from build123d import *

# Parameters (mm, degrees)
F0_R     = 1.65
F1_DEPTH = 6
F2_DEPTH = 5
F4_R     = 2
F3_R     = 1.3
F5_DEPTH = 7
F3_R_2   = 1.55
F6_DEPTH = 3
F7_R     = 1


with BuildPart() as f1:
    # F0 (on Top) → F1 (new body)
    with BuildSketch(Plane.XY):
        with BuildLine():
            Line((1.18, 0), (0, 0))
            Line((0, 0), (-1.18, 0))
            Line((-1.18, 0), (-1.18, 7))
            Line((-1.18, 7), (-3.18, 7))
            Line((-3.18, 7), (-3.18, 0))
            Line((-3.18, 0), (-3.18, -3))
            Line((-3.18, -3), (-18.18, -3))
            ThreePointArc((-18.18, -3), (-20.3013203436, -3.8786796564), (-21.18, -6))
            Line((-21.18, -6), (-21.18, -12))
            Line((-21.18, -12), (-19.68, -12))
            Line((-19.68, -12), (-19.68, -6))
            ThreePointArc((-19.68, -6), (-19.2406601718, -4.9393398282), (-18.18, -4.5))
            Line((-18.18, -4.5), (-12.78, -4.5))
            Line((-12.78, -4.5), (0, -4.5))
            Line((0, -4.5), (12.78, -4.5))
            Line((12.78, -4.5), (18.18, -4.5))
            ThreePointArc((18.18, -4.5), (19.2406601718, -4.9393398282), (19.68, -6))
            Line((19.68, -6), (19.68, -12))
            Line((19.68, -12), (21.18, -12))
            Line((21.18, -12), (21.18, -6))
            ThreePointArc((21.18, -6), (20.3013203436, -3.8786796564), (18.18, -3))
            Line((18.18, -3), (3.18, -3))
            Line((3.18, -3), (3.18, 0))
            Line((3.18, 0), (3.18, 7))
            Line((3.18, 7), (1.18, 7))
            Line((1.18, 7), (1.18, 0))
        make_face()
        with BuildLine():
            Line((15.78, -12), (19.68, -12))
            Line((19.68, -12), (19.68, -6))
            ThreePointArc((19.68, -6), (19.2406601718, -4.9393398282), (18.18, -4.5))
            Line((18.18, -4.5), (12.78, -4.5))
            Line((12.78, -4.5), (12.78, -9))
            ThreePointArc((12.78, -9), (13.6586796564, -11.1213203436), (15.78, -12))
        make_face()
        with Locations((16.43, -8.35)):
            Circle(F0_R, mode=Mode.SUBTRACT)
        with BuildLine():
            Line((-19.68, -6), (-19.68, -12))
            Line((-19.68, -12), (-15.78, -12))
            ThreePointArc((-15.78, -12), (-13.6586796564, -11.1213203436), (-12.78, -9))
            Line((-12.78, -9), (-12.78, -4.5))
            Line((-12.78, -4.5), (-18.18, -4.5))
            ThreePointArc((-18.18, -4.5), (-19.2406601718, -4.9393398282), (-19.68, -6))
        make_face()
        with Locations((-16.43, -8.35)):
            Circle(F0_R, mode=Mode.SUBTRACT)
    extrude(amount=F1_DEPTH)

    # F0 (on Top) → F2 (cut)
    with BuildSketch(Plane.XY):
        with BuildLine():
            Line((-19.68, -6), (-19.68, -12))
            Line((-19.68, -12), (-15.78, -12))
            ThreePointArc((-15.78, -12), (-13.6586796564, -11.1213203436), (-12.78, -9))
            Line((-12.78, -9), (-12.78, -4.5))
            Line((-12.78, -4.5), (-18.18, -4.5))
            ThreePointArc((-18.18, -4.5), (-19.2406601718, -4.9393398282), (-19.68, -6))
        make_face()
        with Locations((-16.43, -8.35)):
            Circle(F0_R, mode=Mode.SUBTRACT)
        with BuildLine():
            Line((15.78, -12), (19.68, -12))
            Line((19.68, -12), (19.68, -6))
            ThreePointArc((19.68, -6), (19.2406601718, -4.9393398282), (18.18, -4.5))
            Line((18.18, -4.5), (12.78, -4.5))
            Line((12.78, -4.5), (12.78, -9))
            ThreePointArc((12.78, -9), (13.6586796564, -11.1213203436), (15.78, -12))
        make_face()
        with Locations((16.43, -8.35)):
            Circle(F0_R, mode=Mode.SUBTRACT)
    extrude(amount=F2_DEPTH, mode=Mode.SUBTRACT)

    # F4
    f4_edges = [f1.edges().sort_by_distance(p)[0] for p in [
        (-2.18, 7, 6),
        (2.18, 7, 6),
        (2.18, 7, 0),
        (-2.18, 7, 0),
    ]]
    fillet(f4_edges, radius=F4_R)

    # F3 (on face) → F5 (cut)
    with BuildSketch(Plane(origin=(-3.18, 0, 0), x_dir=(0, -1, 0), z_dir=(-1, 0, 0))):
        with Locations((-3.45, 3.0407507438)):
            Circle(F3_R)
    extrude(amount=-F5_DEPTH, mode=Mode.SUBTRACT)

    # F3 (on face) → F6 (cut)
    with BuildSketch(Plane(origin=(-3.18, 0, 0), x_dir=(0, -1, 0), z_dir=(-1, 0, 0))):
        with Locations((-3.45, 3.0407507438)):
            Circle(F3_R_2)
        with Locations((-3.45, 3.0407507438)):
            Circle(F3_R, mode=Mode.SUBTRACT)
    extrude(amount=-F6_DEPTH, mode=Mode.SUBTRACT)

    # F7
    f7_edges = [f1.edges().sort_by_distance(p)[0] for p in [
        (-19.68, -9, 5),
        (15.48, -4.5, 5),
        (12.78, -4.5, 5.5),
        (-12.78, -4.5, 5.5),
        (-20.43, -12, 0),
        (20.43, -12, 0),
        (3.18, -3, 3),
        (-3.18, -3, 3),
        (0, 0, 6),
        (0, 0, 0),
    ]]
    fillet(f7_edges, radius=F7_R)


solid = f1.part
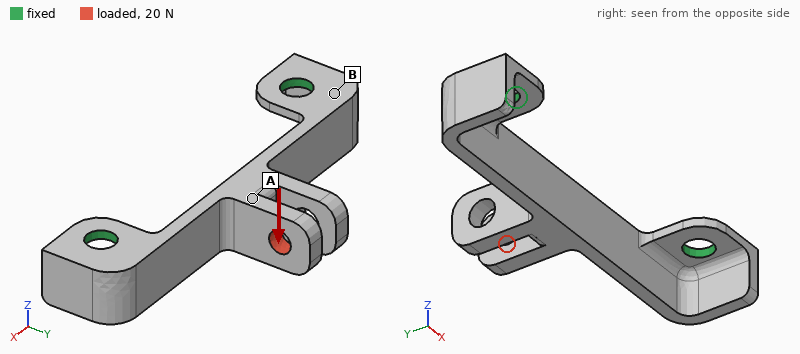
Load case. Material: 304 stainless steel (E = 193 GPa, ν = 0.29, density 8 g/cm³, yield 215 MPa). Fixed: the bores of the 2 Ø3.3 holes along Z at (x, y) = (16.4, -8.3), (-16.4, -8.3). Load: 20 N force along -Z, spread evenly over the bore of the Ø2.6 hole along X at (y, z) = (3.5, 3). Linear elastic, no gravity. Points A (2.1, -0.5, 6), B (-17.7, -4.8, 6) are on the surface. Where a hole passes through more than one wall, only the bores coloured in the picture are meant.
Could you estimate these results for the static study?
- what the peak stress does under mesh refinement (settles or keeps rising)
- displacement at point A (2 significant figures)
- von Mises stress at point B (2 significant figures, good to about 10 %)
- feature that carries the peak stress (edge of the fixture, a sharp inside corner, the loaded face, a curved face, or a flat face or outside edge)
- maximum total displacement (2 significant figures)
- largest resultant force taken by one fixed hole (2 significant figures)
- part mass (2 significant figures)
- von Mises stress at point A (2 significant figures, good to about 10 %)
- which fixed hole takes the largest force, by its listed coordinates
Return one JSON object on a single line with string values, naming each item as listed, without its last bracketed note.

{"what the peak stress does under mesh refinement": "keeps rising", "displacement at point A": "13 µm", "von Mises stress at point B": "20 MPa", "feature that carries the peak stress": "edge of the fixture", "maximum total displacement": "34 µm", "largest resultant force taken by one fixed hole": "16 N", "part mass": "6.7 g", "von Mises stress at point A": "6.3 MPa", "which fixed hole takes the largest force, by its listed coordinates": "(16.4, -8.3)"}
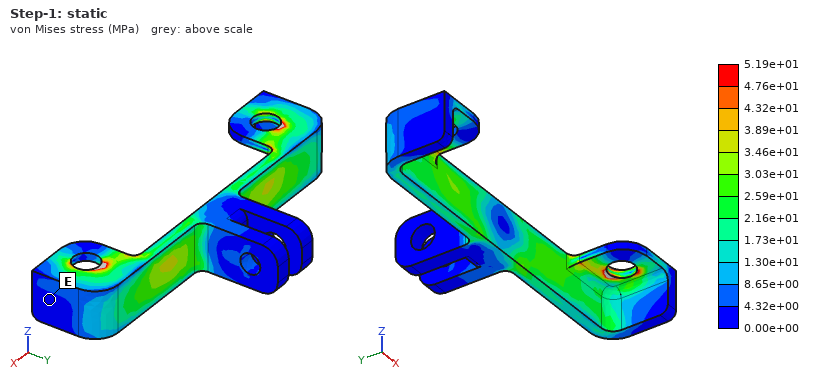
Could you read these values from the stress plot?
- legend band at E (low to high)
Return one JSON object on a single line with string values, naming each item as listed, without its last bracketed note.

{"legend band at E": "0.00e+00 to 4.32e+00 MPa"}
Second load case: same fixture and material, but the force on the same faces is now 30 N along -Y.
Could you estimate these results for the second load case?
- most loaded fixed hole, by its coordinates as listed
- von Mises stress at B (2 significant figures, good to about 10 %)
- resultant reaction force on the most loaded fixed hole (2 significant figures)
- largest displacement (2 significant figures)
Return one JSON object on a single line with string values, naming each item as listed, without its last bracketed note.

{"most loaded fixed hole, by its coordinates as listed": "(16.4, -8.3)", "von Mises stress at B": "10 MPa", "resultant reaction force on the most loaded fixed hole": "23 N", "largest displacement": "14 µm"}
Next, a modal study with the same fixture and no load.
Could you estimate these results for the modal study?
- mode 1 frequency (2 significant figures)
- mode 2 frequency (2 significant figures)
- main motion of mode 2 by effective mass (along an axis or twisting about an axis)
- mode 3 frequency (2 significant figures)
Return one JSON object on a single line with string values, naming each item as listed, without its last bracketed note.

{"mode 1 frequency": "3600 Hz", "mode 2 frequency": "6400 Hz", "main motion of mode 2 by effective mass": "along Y", "mode 3 frequency": "9900 Hz"}
